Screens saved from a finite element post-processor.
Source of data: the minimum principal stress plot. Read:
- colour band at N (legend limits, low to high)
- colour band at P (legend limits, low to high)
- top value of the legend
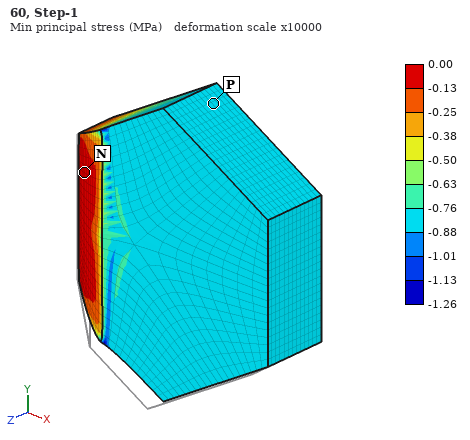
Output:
-0.13 to 0.00 MPa
-0.88 to -0.76 MPa
0.00 MPa
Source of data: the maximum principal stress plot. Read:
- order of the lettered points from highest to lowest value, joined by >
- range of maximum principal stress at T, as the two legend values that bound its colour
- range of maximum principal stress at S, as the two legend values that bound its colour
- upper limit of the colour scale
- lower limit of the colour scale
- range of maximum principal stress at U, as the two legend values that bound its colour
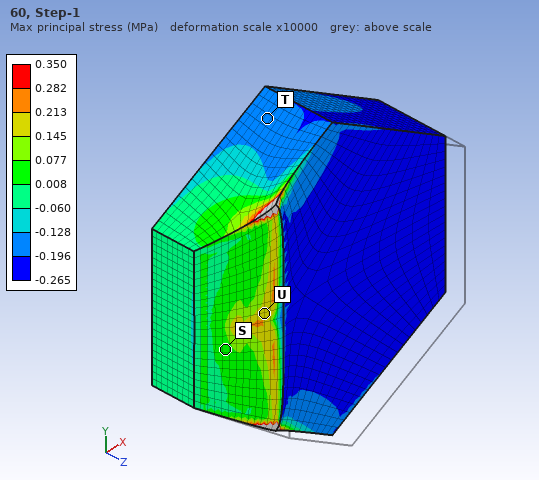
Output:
U > S > T
-0.196 to -0.128 MPa
0.008 to 0.077 MPa
0.350 MPa
-0.265 MPa
0.145 to 0.213 MPa
